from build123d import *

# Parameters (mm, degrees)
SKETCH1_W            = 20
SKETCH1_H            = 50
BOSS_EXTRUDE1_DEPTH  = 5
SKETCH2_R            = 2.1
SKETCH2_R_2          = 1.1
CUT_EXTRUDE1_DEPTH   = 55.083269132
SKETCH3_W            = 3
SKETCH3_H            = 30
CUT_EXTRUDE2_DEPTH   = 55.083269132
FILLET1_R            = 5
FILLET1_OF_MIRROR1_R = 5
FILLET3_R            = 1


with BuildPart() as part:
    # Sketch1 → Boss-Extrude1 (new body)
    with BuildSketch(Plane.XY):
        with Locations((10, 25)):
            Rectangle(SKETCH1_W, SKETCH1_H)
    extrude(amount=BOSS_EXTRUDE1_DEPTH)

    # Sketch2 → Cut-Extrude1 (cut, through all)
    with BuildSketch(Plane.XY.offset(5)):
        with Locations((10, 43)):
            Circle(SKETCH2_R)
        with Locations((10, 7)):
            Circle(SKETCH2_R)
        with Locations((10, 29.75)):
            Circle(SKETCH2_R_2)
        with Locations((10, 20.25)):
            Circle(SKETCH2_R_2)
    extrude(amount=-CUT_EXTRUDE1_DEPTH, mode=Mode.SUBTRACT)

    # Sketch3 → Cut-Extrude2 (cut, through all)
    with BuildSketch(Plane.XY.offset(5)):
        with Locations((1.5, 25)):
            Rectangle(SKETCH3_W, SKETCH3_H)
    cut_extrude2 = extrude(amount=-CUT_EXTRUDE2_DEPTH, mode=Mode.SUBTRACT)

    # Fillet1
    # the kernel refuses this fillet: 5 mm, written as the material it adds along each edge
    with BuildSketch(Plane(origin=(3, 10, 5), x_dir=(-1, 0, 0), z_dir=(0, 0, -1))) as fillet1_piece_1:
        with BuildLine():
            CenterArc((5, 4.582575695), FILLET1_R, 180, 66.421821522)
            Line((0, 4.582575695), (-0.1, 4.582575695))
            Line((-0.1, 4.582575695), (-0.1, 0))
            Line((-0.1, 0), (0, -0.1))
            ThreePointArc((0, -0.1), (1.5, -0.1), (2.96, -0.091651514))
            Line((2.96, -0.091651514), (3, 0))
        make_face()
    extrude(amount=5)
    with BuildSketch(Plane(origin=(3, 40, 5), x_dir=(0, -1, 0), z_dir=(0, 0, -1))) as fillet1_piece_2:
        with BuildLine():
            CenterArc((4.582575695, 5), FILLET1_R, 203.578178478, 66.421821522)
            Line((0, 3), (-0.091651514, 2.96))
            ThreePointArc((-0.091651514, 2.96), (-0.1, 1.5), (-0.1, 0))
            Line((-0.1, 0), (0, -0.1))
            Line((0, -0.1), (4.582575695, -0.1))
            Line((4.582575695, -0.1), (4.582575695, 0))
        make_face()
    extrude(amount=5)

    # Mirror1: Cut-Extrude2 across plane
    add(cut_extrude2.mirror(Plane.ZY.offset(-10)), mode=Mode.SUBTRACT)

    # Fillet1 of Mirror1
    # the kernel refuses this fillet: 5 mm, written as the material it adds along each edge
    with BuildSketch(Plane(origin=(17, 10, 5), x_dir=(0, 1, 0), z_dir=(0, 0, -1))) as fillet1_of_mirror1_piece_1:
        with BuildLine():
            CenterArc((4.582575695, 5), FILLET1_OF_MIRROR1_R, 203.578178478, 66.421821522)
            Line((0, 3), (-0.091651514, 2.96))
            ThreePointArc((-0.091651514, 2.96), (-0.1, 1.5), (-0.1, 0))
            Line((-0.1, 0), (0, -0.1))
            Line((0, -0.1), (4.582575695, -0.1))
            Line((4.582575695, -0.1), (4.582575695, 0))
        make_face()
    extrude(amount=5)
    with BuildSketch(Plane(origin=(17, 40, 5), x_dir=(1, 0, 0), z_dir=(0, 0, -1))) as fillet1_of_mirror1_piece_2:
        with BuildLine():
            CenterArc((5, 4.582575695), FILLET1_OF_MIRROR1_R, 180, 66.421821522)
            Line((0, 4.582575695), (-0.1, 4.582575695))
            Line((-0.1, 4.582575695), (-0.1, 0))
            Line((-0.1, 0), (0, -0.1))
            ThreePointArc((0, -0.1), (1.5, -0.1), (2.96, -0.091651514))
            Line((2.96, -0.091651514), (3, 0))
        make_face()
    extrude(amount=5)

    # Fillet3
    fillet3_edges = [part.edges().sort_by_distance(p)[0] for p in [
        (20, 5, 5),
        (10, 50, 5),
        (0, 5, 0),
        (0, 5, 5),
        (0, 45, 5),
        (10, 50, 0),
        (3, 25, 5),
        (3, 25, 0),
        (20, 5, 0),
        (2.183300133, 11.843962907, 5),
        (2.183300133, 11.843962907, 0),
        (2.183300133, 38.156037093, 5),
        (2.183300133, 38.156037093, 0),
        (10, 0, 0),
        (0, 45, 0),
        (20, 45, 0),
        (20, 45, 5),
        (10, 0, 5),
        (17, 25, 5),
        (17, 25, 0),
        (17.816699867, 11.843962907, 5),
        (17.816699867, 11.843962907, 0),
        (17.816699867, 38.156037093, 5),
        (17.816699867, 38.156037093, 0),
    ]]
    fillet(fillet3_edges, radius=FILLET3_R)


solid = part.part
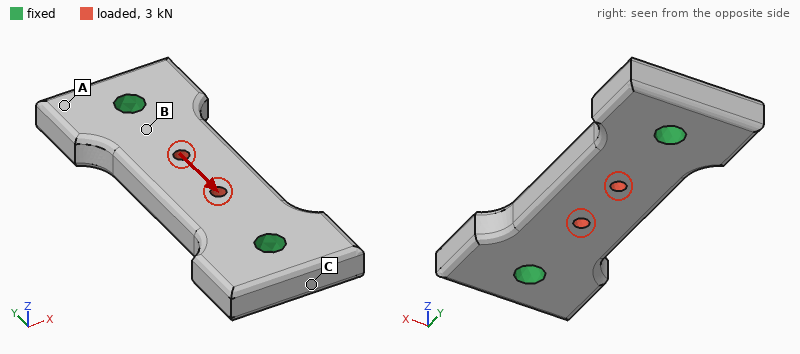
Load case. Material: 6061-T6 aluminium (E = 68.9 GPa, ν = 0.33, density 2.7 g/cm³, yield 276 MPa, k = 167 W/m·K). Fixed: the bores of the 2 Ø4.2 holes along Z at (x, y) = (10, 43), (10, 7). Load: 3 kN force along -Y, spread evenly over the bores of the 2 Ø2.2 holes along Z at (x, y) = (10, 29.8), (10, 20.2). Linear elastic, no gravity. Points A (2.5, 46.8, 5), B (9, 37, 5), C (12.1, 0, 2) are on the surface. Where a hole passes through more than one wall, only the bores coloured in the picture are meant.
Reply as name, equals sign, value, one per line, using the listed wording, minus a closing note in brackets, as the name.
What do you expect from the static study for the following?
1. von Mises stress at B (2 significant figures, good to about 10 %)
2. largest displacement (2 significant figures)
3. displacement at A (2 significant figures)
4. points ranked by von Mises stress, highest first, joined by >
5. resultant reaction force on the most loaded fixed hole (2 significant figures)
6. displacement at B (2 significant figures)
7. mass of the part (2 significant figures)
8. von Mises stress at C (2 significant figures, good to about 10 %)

von Mises stress at B = 33 MPa
largest displacement = 6.6 µm
displacement at A = 1.6 µm
points ranked by von Mises stress, highest first, joined by > = B > C > A
resultant reaction force on the most loaded fixed hole = 1.5 kN
displacement at B = 2.1 µm
mass of the part = 11 g
von Mises stress at C = 11 MPa
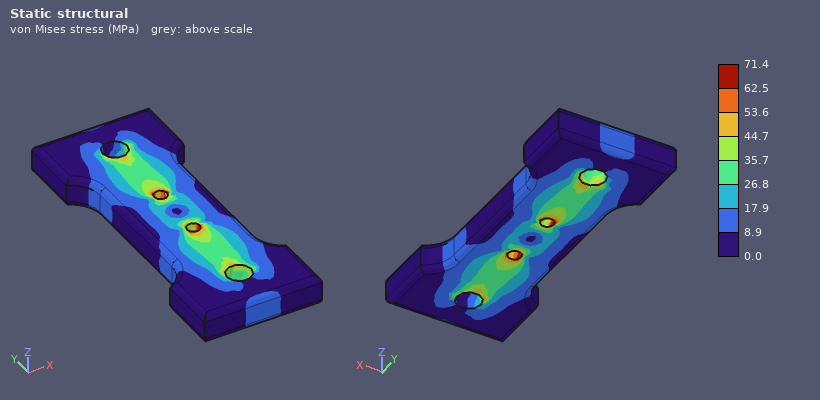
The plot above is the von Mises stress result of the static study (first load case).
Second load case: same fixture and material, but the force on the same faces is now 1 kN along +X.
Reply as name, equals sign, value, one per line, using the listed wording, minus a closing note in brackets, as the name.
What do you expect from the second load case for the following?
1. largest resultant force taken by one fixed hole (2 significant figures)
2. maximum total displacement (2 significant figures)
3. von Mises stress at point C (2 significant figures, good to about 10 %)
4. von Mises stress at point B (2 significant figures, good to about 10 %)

largest resultant force taken by one fixed hole = 500 N
maximum total displacement = 9.0 µm
von Mises stress at point C = 3.3 MPa
von Mises stress at point B = 17 MPa
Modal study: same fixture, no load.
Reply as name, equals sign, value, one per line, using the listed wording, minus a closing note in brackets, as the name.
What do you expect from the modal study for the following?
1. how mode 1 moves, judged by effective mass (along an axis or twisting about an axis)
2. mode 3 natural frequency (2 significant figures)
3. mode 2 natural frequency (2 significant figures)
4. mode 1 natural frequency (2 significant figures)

how mode 1 moves, judged by effective mass = along Z
mode 3 natural frequency = 28 kHz
mode 2 natural frequency = 27 kHz
mode 1 natural frequency = 19 kHz
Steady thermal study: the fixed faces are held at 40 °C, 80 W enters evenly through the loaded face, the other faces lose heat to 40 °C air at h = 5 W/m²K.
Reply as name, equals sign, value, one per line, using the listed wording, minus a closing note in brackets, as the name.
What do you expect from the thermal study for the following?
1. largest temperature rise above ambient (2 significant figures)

largest temperature rise above ambient = 53 K
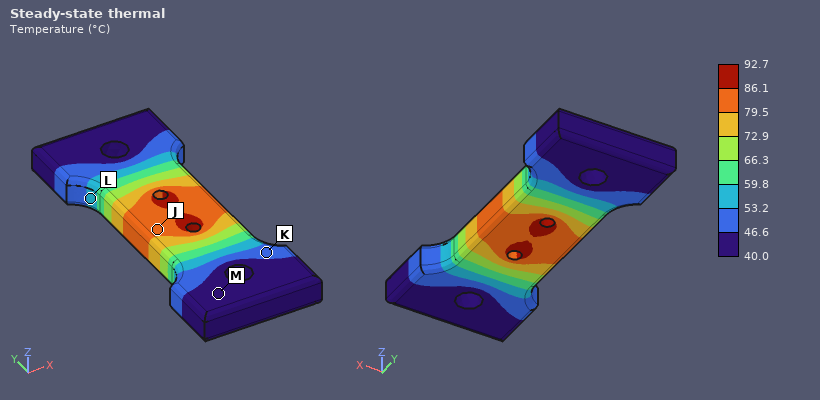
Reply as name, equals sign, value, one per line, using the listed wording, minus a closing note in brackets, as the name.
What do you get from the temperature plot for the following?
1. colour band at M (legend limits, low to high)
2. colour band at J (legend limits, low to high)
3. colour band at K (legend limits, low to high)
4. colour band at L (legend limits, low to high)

colour band at M = 40.0 to 46.6 °C
colour band at J = 79.5 to 86.1 °C
colour band at K = 46.6 to 53.2 °C
colour band at L = 53.2 to 59.8 °C
